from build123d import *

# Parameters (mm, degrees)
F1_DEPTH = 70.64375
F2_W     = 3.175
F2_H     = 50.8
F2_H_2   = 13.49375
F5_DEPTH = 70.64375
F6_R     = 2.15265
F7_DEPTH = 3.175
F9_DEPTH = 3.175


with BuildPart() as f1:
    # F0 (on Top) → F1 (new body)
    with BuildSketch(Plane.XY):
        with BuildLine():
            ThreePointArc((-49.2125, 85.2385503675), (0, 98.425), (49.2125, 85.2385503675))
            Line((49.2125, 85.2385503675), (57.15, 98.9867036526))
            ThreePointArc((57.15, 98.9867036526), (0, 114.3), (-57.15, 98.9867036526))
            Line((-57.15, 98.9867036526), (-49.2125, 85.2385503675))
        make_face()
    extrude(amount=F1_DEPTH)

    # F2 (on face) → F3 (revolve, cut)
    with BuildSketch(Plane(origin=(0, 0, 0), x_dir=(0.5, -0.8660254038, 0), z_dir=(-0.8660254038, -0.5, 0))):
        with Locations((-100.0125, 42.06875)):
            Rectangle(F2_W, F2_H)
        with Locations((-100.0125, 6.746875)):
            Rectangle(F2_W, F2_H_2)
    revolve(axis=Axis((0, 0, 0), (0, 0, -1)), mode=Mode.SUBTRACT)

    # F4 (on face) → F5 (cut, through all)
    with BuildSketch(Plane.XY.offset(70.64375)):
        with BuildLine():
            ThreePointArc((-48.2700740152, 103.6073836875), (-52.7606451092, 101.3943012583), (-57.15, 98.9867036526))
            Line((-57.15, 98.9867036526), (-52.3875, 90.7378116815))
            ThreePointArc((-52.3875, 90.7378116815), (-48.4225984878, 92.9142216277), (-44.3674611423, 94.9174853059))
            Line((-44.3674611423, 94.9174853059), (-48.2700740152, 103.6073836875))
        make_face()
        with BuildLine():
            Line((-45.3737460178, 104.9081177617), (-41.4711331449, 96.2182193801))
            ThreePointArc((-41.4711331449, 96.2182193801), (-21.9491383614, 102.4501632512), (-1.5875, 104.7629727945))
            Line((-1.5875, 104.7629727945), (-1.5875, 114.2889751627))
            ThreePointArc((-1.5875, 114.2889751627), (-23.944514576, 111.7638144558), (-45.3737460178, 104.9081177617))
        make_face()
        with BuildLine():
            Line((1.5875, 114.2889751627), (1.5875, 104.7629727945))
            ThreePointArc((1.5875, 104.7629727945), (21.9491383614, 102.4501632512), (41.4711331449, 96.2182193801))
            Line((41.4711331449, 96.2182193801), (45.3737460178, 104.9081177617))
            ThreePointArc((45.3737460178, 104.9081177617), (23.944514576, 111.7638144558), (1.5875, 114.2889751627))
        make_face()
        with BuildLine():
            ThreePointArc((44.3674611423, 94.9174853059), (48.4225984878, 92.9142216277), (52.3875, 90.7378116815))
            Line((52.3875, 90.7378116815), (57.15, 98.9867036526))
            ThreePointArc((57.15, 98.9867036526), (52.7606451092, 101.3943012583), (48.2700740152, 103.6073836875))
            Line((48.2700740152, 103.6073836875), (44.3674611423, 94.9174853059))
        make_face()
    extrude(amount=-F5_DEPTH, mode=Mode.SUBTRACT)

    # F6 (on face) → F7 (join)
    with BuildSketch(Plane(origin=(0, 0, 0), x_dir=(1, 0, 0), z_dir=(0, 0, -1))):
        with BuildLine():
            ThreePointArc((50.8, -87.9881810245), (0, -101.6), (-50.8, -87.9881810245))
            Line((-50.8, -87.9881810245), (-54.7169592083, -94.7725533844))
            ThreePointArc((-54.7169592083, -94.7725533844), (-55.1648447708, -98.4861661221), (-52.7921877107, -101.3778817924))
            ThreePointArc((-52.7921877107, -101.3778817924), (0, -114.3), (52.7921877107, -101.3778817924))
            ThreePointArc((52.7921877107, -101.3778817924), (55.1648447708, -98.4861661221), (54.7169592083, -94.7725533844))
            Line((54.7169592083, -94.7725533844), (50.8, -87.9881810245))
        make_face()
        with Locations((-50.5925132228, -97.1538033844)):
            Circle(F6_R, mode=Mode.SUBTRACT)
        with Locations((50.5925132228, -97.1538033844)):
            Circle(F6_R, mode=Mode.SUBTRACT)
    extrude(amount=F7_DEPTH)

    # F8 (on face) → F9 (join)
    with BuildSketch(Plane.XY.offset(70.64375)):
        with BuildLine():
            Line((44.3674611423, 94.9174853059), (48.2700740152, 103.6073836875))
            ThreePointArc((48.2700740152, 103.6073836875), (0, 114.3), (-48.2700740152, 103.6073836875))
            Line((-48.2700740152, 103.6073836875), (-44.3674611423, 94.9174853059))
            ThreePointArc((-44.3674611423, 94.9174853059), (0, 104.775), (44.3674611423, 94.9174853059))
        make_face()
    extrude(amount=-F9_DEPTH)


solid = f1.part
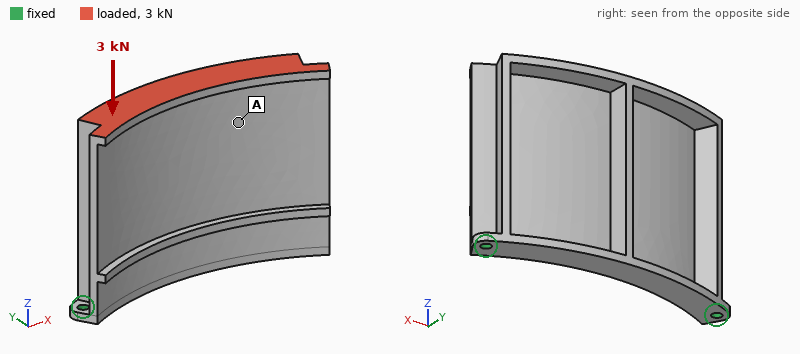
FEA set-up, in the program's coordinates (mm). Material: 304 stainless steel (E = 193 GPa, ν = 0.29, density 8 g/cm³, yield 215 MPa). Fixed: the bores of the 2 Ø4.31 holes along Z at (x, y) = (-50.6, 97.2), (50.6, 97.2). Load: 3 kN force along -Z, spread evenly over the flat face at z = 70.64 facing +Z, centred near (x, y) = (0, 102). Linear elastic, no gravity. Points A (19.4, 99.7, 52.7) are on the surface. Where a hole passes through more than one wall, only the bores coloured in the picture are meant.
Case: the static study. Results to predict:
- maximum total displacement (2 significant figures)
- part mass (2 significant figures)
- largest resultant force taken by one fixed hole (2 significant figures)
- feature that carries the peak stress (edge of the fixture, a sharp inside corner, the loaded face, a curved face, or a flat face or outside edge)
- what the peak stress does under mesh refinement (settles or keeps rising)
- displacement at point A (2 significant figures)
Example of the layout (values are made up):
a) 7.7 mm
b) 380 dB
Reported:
a) 0.22 mm
b) 320 g
c) 1.7 kN
d) edge of the fixture
e) keeps rising
f) 0.15 mm
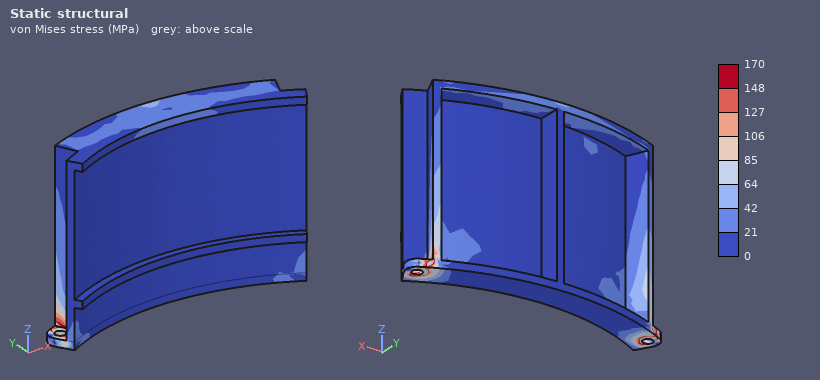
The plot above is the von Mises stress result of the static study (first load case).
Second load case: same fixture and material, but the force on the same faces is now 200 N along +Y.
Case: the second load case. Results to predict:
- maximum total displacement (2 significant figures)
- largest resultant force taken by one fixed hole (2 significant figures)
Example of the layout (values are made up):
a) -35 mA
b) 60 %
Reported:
a) 0.15 mm
b) 100 N
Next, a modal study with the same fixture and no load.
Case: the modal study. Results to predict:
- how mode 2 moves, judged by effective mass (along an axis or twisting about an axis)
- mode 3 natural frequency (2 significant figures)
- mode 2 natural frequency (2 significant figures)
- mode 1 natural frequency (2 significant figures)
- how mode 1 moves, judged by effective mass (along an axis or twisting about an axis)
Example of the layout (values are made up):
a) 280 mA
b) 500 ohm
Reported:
a) twisting about Z
b) 3600 Hz
c) 1000 Hz
d) 560 Hz
e) along Y
